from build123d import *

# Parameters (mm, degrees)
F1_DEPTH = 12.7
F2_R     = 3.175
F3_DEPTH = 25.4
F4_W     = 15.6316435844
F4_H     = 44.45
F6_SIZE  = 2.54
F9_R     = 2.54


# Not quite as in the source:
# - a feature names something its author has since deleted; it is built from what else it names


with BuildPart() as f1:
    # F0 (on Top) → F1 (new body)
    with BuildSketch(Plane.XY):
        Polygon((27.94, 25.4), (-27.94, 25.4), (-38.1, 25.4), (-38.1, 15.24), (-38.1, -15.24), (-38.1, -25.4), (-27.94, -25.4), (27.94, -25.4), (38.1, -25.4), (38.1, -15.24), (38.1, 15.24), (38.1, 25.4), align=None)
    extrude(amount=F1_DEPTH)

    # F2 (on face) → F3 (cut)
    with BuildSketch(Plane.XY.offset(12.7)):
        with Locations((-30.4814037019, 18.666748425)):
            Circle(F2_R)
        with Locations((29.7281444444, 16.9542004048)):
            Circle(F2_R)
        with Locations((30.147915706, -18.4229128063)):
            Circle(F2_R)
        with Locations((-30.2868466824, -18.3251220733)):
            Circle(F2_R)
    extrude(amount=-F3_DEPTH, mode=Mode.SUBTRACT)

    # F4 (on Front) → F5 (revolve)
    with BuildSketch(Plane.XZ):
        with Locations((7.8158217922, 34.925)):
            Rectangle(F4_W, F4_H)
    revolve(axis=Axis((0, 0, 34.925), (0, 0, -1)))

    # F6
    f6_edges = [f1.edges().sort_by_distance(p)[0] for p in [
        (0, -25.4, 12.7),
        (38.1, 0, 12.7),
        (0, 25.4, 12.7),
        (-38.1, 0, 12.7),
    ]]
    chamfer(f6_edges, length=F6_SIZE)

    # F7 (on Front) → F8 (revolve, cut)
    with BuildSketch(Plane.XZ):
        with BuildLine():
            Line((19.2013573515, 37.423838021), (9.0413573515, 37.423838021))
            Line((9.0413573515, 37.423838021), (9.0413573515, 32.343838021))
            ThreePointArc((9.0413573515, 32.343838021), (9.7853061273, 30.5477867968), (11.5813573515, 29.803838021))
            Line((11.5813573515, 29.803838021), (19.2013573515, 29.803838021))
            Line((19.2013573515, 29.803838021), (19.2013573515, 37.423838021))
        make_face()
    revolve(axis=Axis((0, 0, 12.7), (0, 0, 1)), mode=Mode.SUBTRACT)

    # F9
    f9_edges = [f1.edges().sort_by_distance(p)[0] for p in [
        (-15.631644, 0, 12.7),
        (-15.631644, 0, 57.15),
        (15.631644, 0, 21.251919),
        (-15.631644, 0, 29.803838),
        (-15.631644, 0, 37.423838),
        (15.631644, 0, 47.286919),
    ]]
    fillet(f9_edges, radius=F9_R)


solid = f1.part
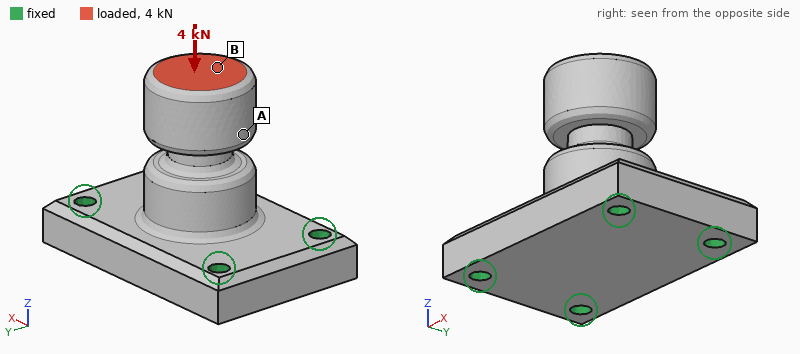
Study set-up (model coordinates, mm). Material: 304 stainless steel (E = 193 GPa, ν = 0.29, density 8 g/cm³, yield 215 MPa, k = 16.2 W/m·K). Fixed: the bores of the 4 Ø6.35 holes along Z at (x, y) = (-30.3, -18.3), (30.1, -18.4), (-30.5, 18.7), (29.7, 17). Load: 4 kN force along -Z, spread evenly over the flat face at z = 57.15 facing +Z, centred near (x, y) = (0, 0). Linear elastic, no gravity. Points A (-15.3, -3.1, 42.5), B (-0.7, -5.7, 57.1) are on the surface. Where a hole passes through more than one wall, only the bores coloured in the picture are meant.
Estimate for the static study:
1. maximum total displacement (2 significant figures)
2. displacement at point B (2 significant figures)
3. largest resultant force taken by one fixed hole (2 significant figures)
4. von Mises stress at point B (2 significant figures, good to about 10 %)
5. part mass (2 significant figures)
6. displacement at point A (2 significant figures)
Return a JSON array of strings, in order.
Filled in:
["4.8 µm", "4.8 µm", "1.1 kN", "5.9 MPa", "610 g", "4.5 µm"]
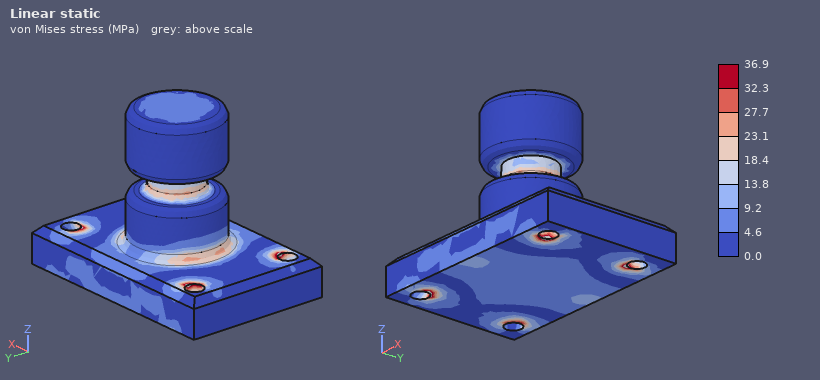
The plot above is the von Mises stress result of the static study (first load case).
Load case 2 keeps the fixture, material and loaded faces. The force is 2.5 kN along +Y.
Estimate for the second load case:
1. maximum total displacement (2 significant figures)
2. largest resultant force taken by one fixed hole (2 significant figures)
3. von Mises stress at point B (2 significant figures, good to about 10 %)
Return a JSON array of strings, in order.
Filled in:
["45 µm", "1.9 kN", "8.7 MPa"]
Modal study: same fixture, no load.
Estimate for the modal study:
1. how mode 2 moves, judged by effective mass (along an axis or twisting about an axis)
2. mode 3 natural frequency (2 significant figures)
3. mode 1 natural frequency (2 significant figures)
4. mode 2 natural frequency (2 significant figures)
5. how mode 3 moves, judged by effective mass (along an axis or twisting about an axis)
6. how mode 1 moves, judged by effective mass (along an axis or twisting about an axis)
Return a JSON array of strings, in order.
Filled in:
["along X", "9200 Hz", "4400 Hz", "5100 Hz", "along Z", "along Y"]
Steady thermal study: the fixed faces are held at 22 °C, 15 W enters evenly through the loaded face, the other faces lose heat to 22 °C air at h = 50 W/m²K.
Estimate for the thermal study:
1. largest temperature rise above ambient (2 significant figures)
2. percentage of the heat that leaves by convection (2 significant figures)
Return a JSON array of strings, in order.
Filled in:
["64 K", "63 %"]
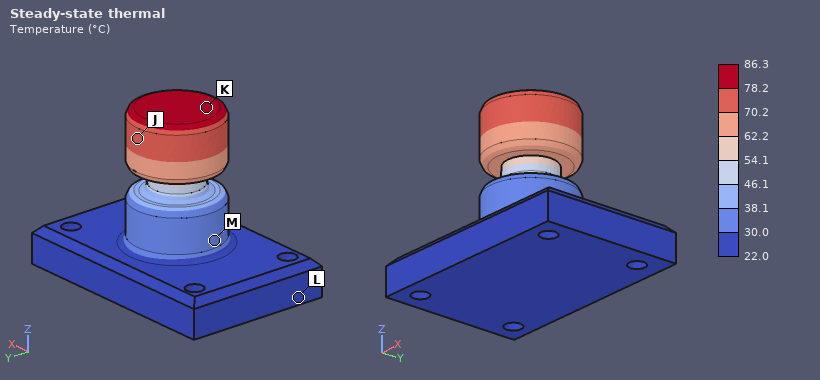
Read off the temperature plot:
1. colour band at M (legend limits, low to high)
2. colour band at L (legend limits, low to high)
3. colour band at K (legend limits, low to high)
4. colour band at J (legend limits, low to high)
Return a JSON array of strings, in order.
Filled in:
["30.0 to 38.1 °C", "22.0 to 30.0 °C", "78.2 to 86.3 °C", "70.2 to 78.2 °C"]
